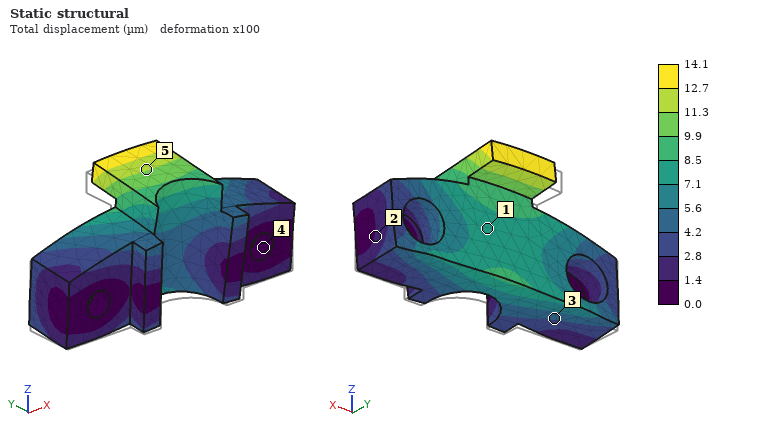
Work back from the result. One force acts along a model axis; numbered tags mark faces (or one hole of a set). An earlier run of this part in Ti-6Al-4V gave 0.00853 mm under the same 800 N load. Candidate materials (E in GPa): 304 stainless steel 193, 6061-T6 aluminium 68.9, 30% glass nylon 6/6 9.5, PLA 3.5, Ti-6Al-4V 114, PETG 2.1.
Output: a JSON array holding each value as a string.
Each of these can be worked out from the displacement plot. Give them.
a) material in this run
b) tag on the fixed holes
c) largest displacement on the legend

["6061-T6 aluminium", "4", "14.1 µm"]
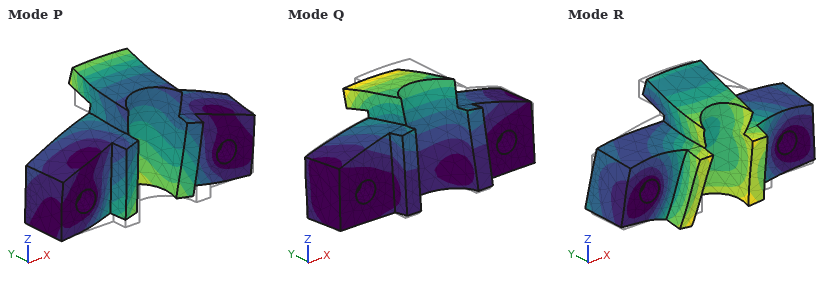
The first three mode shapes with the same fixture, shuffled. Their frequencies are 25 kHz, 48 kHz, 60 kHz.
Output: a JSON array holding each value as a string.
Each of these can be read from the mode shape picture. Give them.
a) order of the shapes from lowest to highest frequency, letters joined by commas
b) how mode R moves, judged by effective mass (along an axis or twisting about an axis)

["Q, P, R", "along Z"]
